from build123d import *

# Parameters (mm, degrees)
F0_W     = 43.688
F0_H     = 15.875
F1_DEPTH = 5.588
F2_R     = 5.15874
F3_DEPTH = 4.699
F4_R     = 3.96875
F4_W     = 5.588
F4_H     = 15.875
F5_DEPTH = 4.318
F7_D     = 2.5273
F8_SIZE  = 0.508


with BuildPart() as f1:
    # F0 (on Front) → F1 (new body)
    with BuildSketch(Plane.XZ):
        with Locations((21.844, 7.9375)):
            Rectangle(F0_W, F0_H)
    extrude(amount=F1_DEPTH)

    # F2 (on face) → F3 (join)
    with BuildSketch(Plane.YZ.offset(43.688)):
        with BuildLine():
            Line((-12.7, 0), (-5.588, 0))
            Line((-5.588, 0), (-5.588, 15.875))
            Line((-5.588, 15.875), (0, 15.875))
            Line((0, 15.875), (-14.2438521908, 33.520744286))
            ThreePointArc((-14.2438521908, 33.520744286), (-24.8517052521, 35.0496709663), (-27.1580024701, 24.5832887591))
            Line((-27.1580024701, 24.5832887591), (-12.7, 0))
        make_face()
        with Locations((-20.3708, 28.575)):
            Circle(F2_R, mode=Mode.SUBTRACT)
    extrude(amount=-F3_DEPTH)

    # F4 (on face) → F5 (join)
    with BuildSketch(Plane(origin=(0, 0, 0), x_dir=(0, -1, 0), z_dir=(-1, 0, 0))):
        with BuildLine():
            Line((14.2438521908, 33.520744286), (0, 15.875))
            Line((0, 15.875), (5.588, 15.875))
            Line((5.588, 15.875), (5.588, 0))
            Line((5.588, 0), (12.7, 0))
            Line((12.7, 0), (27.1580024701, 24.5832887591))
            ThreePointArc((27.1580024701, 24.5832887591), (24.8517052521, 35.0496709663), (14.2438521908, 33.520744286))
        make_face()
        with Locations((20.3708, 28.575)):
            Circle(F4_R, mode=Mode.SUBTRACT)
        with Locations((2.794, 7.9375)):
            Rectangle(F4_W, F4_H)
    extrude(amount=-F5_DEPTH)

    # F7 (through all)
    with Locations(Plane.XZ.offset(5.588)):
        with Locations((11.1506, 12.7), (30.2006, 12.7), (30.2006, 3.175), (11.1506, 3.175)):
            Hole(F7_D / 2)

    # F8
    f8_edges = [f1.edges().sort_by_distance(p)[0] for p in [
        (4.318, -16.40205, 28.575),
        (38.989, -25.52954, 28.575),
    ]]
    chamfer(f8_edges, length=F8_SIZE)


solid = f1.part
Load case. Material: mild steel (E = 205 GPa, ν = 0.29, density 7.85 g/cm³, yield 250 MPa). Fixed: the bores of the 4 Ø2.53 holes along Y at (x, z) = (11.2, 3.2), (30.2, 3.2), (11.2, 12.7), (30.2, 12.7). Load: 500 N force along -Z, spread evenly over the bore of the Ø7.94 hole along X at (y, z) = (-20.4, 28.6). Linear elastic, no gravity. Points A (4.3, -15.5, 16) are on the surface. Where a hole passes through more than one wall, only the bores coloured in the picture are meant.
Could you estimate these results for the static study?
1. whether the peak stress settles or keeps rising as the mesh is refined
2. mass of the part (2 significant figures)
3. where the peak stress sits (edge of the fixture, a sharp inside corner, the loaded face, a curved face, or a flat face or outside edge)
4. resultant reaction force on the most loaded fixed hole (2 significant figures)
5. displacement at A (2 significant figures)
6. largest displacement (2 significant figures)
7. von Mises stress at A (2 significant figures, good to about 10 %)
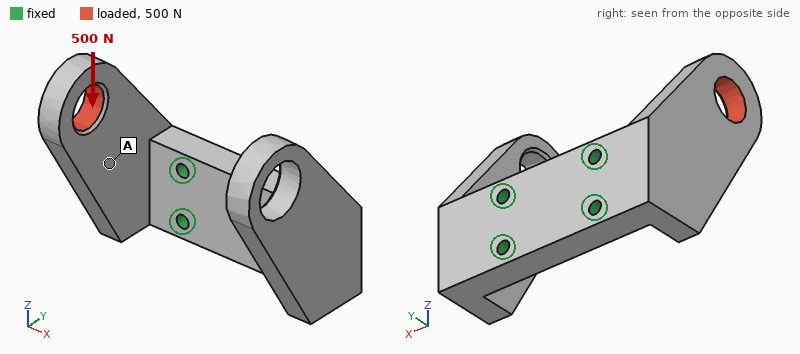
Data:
keeps rising
64 g
edge of the fixture
820 N
14 µm
35 µm
11 MPa
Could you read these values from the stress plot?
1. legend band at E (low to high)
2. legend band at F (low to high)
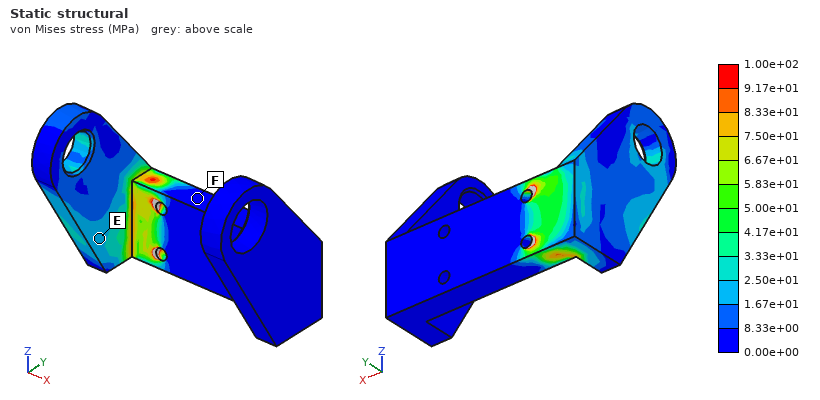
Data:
1.67e+01 to 2.50e+01 MPa
0.00e+00 to 8.33e+00 MPa
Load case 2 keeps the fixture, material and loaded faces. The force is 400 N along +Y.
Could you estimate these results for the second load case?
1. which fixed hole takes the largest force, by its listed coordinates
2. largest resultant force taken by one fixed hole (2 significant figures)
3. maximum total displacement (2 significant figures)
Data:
(11.2, 12.7)
850 N
40 µm
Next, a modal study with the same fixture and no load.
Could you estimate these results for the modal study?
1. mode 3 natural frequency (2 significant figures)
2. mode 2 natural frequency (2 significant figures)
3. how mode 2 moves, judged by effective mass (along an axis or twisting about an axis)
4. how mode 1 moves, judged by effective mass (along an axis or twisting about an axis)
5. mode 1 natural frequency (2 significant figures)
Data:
5800 Hz
3900 Hz
along X
along X
3700 Hz
